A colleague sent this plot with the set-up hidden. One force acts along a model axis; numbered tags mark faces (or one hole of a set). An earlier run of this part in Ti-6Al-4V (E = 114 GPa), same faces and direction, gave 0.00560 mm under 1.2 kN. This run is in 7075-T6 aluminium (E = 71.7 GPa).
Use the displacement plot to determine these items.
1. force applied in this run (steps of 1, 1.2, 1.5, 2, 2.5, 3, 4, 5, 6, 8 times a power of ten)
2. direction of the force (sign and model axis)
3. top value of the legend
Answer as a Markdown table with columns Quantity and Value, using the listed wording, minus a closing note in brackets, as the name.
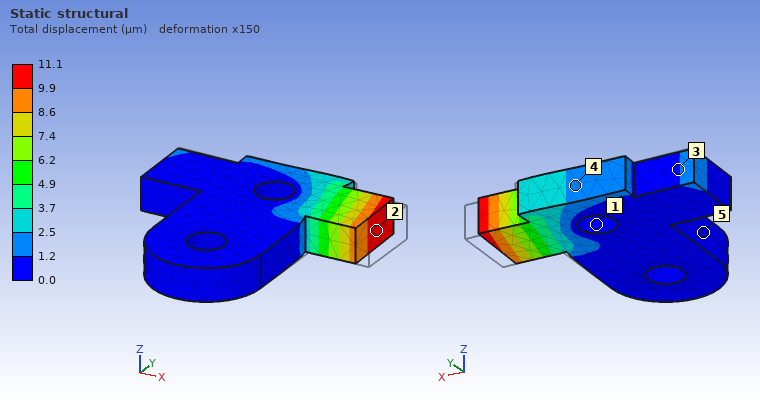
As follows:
| Quantity | Value |
|---|---|
| force applied in this run | 1.5 kN |
| direction of the force | -X |
| top value of the legend | 11.1 µm |
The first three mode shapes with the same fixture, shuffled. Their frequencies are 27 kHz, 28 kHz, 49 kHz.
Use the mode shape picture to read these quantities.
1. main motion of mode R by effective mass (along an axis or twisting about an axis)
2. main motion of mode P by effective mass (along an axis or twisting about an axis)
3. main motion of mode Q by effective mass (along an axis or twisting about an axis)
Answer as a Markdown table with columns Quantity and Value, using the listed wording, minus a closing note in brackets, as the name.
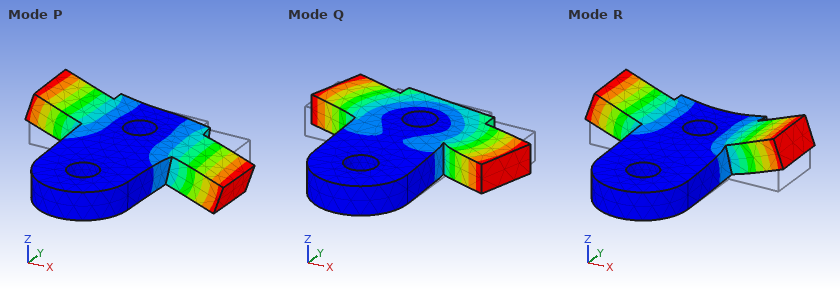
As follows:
| Quantity | Value |
|---|---|
| main motion of mode R by effective mass | along Z |
| main motion of mode P by effective mass | twisting about Y |
| main motion of mode Q by effective mass | twisting about Z |
